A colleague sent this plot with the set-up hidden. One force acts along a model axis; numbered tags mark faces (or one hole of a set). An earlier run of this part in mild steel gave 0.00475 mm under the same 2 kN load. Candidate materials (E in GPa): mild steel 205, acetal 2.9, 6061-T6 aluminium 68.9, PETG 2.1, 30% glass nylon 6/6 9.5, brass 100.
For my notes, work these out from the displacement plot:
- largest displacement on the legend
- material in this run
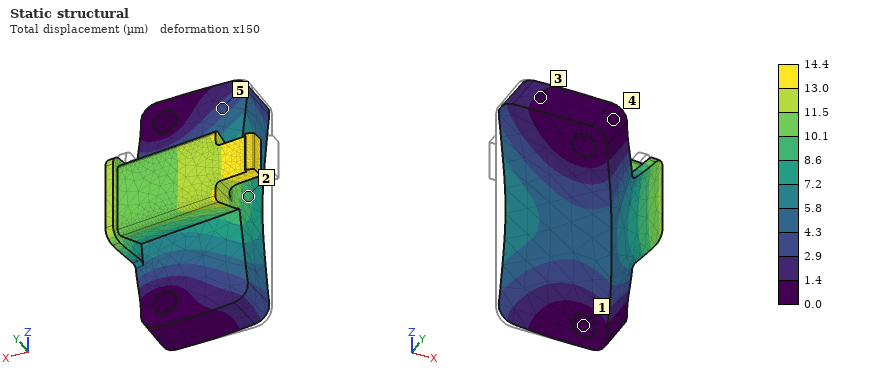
14.4 µm
6061-T6 aluminium
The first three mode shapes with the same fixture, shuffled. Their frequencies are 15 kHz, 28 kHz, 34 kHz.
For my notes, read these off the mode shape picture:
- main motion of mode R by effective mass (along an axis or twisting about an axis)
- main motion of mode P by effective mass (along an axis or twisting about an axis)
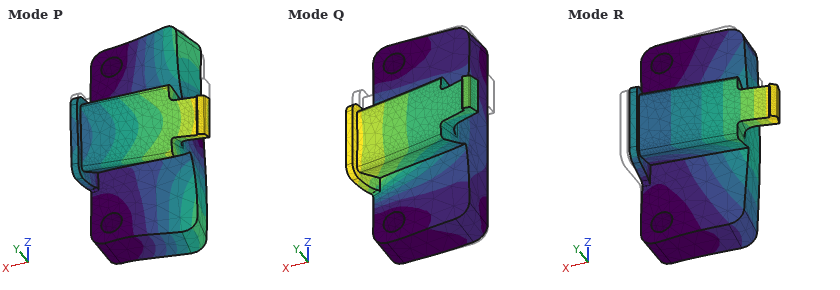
along Y
along Z
